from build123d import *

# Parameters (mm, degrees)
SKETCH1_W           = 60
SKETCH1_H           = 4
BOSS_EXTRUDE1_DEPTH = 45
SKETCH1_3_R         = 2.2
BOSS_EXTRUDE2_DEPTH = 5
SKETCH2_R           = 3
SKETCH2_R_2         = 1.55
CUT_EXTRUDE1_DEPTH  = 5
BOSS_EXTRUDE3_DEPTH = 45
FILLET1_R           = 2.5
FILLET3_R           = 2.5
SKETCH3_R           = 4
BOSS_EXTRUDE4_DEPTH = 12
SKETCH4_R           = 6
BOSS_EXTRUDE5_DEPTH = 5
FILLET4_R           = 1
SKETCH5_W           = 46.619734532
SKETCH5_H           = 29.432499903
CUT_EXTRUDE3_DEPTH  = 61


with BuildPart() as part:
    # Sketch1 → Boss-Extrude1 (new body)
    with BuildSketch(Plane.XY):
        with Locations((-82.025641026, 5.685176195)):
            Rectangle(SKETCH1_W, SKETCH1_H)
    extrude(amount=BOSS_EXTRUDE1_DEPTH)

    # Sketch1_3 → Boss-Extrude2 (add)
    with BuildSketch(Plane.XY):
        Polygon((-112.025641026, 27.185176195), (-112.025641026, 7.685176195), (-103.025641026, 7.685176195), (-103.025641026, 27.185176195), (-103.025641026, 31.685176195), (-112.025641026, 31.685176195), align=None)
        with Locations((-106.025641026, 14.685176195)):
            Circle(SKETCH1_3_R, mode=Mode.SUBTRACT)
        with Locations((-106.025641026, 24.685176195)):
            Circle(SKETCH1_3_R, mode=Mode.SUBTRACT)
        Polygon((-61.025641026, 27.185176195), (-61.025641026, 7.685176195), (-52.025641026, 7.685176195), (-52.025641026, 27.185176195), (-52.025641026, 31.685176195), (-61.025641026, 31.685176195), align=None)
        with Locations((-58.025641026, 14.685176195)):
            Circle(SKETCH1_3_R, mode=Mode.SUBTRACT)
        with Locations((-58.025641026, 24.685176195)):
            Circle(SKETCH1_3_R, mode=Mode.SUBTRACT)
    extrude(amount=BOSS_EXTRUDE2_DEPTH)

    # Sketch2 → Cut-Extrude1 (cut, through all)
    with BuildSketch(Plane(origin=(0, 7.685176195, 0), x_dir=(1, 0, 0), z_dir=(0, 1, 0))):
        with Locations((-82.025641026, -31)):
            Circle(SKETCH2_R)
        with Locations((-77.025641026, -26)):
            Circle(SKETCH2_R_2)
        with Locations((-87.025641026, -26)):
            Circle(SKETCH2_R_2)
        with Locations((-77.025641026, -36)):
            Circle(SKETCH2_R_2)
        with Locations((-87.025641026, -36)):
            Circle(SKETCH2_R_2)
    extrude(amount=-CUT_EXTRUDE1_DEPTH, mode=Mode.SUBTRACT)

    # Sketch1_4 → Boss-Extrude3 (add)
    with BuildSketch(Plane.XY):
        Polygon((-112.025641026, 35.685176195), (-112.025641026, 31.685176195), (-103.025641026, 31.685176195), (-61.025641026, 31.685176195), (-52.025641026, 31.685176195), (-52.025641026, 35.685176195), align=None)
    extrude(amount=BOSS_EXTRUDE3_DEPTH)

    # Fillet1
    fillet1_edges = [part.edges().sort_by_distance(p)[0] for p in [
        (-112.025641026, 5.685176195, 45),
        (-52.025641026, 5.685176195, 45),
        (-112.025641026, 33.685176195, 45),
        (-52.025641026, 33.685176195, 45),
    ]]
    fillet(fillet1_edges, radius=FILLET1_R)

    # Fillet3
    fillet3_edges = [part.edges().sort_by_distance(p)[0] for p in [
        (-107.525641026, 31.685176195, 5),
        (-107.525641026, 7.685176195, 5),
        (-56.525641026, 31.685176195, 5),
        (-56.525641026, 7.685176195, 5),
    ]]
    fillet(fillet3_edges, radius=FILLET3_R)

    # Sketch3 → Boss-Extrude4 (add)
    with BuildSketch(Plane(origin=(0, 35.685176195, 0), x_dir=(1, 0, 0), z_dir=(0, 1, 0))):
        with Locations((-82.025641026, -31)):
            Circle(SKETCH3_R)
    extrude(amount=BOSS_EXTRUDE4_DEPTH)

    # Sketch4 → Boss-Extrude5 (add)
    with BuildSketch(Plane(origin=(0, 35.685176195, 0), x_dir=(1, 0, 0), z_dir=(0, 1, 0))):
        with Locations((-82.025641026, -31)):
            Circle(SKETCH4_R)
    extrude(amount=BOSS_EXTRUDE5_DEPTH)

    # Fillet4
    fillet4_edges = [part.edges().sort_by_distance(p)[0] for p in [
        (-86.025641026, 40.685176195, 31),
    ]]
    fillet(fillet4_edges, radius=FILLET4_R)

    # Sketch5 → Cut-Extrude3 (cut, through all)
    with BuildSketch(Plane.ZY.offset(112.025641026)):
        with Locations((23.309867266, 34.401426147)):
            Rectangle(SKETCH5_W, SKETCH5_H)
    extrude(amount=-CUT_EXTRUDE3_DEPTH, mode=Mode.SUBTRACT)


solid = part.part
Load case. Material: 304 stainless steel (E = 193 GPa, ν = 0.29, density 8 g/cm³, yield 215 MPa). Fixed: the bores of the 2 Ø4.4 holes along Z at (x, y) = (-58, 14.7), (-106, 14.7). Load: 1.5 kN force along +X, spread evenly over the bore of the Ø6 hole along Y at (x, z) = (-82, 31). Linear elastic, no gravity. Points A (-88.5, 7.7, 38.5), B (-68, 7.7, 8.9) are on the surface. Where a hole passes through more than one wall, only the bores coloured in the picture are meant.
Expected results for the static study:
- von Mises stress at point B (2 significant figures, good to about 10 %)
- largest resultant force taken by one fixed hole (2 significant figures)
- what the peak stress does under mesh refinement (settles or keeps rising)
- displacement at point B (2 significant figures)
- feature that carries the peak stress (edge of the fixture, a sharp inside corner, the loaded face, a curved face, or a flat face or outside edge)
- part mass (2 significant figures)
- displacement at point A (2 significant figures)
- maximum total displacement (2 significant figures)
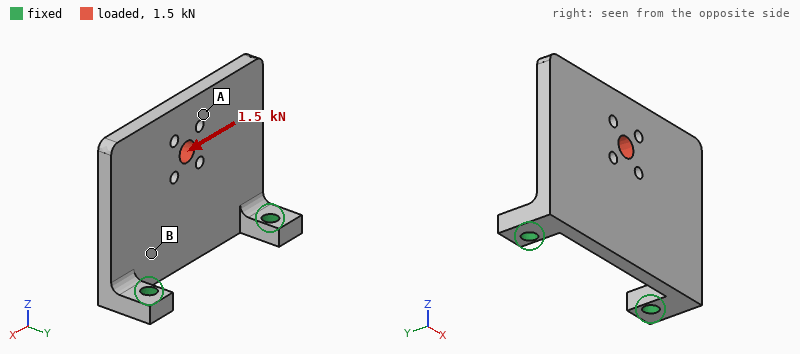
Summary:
31 MPa
1.1 kN
keeps rising
9.1 µm
edge of the fixture
92 g
20 µm
28 µm
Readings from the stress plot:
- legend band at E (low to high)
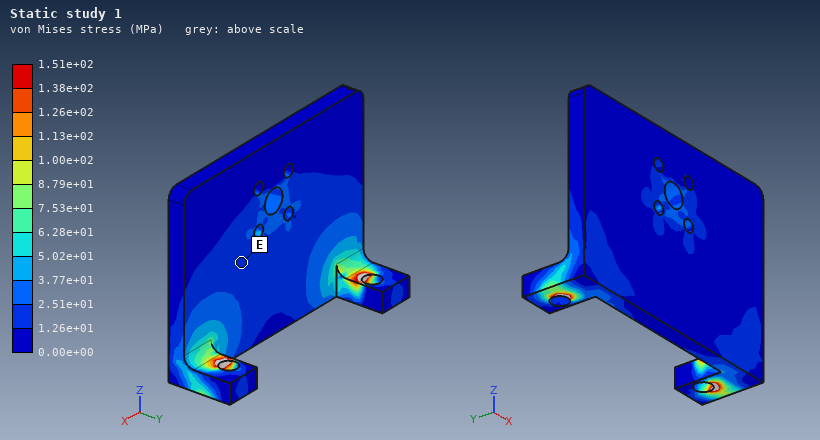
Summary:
1.26e+01 to 2.51e+01 MPa
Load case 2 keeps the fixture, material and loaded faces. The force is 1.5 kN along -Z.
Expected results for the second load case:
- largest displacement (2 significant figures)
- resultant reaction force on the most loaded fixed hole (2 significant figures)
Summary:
57 µm
760 N
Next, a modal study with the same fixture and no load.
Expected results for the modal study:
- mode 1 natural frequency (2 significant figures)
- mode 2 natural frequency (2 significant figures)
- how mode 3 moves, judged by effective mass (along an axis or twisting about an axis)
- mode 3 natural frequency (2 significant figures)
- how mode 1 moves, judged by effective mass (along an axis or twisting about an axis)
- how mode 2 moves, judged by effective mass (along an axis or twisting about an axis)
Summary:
1100 Hz
3000 Hz
along X
6200 Hz
along Y
twisting about Z
